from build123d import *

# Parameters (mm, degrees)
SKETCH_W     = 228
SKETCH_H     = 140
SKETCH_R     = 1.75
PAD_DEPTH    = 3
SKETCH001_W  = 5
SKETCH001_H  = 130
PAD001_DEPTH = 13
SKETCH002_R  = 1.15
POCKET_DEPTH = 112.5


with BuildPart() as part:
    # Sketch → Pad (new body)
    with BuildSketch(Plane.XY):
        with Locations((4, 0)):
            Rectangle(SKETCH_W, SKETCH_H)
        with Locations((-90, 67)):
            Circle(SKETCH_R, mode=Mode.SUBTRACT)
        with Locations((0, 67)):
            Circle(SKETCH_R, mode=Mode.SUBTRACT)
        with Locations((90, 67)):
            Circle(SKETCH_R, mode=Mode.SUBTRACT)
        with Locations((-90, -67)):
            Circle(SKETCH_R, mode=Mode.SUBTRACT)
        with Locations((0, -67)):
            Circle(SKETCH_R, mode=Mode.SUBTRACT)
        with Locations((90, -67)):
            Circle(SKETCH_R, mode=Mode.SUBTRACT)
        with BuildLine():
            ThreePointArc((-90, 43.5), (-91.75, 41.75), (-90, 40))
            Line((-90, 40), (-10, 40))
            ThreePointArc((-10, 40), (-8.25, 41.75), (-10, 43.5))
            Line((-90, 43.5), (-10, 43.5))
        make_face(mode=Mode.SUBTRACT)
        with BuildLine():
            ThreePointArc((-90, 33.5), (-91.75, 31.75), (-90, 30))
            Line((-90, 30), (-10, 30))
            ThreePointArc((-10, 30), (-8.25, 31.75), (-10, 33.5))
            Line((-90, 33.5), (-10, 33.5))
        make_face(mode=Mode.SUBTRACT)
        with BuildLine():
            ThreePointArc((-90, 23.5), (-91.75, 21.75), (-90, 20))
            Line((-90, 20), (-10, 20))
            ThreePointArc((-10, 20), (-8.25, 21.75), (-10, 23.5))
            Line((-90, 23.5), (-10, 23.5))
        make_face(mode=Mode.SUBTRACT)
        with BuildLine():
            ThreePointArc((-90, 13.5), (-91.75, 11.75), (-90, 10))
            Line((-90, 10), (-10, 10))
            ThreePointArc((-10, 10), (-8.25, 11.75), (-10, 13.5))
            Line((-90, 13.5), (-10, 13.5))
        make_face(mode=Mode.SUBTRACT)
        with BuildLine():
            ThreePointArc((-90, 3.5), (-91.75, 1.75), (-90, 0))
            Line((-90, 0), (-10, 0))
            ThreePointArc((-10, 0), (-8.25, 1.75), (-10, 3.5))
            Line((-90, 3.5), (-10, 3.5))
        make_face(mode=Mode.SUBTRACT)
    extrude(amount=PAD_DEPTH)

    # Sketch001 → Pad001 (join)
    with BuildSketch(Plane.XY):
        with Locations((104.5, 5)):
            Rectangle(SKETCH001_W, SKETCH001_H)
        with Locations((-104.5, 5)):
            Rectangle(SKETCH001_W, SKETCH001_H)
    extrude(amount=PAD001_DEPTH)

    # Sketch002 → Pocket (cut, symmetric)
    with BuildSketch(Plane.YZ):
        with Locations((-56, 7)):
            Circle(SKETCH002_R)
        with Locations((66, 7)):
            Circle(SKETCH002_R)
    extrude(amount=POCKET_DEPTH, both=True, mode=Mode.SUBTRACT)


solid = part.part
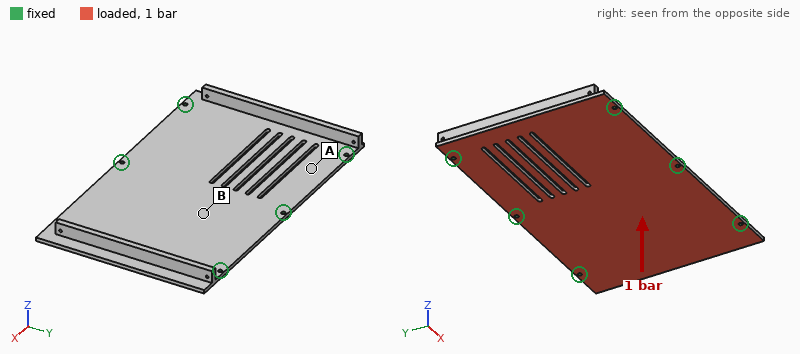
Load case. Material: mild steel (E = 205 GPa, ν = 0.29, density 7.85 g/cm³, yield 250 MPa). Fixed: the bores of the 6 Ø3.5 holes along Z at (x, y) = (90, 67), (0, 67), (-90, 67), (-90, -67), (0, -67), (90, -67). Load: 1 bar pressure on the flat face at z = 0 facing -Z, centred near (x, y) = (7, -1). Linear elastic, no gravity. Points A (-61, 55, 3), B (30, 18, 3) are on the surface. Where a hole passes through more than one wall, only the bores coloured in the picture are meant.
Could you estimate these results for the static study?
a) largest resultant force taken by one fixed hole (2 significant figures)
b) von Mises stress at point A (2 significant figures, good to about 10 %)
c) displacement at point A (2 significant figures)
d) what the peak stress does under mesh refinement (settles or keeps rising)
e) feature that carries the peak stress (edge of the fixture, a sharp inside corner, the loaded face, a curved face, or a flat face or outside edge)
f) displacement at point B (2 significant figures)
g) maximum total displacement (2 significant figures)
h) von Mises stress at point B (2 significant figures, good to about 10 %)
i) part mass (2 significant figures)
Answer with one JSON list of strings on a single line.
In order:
["710 N", "22 MPa", "0.066 mm", "keeps rising", "edge of the fixture", "0.26 mm", "0.38 mm", "49 MPa", "820 g"]
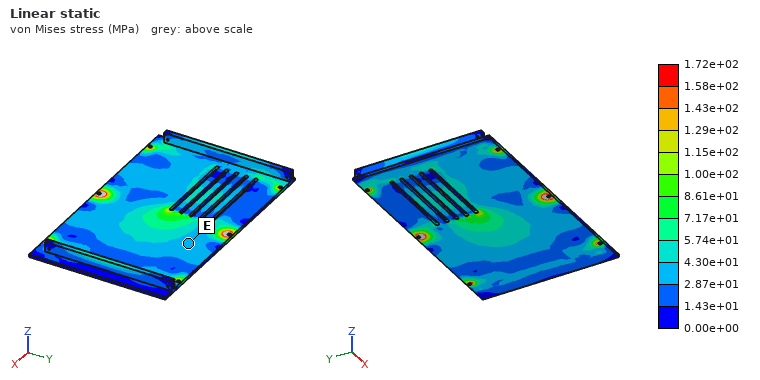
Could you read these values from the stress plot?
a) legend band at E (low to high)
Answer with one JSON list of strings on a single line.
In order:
["2.87e+01 to 4.30e+01 MPa"]
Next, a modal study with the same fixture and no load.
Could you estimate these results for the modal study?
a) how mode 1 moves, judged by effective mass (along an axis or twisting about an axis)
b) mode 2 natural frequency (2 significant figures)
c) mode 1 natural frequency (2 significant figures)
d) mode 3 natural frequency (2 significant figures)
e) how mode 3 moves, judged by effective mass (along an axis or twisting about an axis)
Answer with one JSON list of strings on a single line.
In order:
["along Z", "990 Hz", "690 Hz", "1300 Hz", "along Z"]
